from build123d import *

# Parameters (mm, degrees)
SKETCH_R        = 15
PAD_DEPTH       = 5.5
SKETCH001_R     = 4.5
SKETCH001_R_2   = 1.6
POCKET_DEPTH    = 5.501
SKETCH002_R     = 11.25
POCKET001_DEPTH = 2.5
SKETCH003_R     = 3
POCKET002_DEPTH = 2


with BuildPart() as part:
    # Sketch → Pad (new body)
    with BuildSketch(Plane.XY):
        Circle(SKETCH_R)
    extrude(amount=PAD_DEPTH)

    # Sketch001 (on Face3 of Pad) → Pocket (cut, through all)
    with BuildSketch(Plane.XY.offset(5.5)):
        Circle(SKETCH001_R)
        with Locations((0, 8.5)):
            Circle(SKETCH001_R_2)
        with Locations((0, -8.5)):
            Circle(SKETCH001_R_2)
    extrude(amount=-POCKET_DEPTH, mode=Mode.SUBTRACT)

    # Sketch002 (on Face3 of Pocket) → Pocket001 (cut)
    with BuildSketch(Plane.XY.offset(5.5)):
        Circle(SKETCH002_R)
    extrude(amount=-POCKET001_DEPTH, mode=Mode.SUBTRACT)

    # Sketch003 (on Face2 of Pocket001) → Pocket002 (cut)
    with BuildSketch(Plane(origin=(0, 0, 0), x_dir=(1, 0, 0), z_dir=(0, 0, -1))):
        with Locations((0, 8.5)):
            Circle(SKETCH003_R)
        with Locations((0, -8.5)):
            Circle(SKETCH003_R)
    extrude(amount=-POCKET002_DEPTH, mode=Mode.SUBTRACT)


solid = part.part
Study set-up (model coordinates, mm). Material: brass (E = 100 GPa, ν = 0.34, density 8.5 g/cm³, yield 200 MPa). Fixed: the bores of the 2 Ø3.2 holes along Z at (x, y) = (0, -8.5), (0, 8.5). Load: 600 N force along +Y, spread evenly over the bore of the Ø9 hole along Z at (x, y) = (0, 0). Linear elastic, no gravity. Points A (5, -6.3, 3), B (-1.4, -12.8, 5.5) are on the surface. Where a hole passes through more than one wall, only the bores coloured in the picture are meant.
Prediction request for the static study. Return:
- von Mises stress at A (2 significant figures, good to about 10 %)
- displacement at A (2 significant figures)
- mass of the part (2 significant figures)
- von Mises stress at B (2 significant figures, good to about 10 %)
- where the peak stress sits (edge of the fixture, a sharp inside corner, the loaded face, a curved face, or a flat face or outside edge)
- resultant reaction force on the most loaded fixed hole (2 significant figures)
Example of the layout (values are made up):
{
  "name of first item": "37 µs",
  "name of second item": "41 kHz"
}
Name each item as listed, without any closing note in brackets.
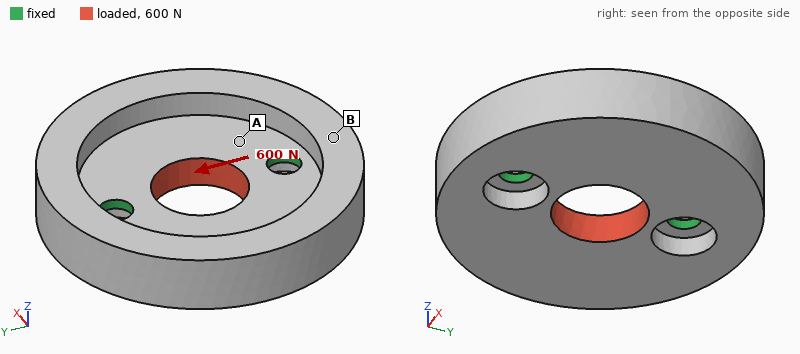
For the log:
{
  "von Mises stress at A": "7.4 MPa",
  "displacement at A": "0.96 µm",
  "mass of the part": "22 g",
  "von Mises stress at B": "3.7 MPa",
  "where the peak stress sits": "edge of the fixture",
  "resultant reaction force on the most loaded fixed hole": "300 N"
}
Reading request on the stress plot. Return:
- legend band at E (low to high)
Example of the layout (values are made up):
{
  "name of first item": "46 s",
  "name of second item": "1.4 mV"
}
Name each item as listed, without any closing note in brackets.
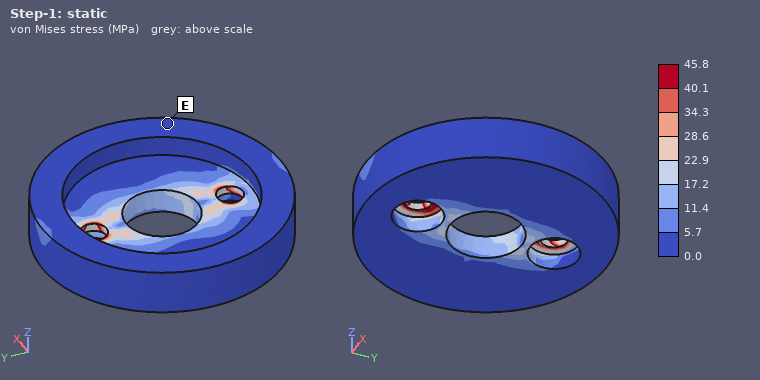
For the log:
{
  "legend band at E": "0.0 to 5.7 MPa"
}
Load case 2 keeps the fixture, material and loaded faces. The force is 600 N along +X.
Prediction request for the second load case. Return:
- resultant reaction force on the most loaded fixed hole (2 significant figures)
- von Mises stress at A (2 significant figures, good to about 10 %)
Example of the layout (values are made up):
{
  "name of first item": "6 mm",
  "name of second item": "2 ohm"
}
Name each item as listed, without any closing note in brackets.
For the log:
{
  "resultant reaction force on the most loaded fixed hole": "300 N",
  "von Mises stress at A": "15 MPa"
}
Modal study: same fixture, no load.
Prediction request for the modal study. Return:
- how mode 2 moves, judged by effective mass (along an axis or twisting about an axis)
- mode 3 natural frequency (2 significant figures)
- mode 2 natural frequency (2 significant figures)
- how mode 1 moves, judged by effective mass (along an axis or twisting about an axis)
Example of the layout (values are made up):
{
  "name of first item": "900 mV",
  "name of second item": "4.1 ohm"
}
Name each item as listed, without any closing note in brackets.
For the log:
{
  "how mode 2 moves, judged by effective mass": "along Z",
  "mode 3 natural frequency": "12 kHz",
  "mode 2 natural frequency": "8200 Hz",
  "how mode 1 moves, judged by effective mass": "twisting about Y"
}
